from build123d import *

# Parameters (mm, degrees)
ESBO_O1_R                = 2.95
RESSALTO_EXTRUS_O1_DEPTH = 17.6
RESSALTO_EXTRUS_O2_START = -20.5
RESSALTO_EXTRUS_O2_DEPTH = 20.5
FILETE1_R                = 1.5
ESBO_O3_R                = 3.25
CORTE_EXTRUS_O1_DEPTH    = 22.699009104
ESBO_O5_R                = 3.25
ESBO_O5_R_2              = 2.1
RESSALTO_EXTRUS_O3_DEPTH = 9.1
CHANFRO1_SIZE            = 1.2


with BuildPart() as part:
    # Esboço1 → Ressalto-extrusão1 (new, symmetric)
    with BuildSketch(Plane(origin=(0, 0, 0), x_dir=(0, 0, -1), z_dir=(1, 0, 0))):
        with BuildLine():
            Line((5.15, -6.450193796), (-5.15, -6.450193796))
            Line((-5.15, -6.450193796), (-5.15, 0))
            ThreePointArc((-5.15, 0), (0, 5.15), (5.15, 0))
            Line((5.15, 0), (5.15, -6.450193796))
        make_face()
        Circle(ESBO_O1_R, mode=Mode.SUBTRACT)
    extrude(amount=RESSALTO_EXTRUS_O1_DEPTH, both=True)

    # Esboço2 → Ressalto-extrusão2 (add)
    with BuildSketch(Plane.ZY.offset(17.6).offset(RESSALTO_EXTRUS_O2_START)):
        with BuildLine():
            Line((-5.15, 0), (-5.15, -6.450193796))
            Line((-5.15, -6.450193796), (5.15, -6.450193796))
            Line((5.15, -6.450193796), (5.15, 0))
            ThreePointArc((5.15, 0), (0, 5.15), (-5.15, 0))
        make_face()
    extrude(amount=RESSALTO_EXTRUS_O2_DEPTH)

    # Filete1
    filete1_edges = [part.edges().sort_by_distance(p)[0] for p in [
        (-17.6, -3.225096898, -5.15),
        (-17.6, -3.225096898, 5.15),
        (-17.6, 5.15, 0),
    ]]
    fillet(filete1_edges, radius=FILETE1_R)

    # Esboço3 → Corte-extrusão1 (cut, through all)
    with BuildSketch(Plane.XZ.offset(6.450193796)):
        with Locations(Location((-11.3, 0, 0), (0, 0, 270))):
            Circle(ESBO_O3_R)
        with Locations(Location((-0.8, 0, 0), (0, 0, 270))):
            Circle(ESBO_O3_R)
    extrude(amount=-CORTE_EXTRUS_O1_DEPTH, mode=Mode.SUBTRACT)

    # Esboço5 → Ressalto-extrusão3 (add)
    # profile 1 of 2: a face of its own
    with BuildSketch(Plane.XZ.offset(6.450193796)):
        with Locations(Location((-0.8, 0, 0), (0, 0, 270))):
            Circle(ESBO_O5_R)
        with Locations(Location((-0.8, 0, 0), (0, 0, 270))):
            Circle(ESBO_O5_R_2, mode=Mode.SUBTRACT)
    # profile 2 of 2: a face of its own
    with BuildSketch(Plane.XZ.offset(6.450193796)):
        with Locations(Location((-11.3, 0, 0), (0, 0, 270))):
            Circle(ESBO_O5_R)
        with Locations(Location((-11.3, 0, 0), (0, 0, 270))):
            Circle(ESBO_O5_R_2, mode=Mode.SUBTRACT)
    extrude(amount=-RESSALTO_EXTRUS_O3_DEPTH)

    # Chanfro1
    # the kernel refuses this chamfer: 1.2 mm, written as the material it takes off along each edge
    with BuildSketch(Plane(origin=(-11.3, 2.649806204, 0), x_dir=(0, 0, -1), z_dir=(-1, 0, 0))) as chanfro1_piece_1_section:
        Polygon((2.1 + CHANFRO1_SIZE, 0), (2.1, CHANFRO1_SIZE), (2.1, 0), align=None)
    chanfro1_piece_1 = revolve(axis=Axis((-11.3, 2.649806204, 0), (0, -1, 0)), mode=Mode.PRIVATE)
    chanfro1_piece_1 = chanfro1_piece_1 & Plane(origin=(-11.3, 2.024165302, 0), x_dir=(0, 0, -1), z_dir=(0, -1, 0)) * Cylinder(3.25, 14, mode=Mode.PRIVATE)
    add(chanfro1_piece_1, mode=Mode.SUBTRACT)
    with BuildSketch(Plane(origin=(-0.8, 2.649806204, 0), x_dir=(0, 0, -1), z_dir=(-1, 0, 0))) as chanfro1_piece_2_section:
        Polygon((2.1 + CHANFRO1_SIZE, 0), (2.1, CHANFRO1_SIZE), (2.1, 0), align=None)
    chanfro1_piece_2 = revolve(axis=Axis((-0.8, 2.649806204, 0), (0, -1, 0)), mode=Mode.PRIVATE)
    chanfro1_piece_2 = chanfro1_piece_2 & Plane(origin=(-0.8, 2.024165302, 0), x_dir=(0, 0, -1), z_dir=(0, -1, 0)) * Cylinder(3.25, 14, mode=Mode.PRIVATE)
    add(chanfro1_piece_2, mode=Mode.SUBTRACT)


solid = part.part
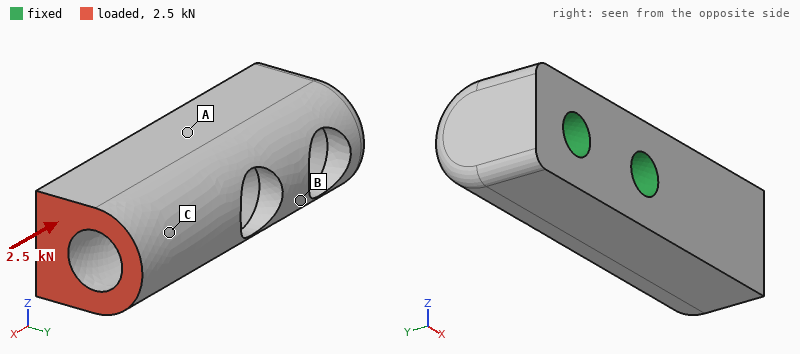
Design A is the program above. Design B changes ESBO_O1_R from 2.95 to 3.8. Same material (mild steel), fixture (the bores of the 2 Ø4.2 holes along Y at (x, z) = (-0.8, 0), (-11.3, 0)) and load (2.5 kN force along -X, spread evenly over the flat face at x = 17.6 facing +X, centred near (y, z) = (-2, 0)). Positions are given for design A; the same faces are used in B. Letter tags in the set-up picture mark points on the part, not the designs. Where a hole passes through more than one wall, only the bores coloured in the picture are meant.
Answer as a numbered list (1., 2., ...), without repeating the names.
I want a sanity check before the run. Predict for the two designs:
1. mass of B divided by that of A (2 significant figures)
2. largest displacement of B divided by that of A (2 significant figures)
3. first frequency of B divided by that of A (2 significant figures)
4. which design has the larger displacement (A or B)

1. 0.91
2. 1.2
3. 1.0
4. B
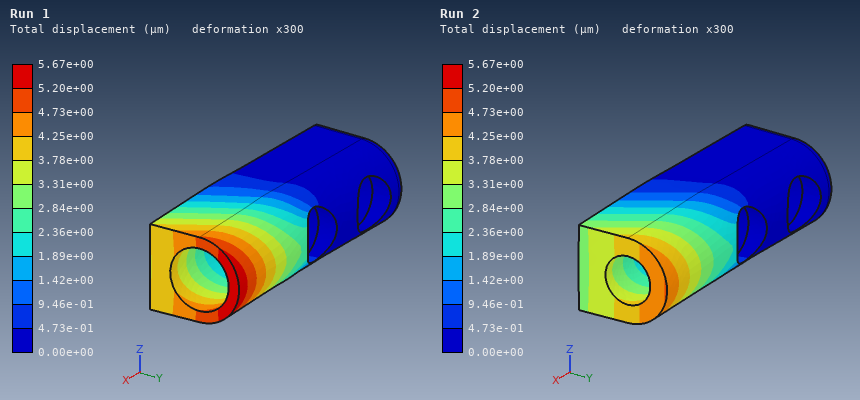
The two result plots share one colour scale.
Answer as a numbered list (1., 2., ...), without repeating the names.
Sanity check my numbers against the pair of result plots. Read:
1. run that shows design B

1. Run 1
